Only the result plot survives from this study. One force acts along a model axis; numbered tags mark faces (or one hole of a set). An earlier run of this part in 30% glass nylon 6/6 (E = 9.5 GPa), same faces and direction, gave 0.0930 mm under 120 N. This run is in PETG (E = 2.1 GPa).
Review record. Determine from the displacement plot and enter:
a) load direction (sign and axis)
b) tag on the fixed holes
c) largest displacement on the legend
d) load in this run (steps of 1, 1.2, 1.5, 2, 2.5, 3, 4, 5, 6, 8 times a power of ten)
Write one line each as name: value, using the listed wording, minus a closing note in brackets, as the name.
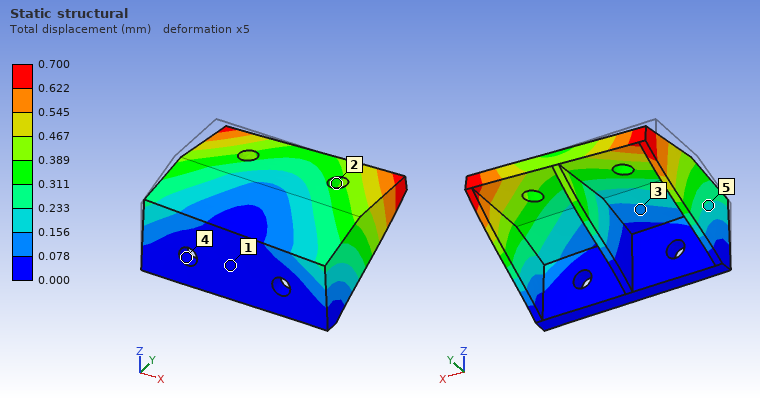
load direction: +X
tag on the fixed holes: 4
largest displacement on the legend: 0.700 mm
load in this run: 200 N
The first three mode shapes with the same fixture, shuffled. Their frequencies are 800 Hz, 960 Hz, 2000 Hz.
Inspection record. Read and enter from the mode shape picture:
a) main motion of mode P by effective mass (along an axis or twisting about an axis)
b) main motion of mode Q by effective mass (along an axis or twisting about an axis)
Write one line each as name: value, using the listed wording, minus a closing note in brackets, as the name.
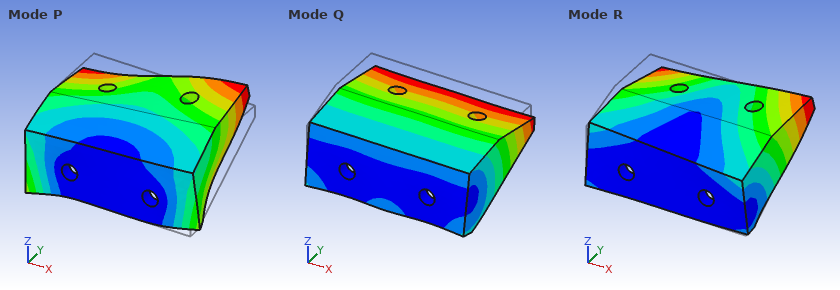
main motion of mode P by effective mass: along X
main motion of mode Q by effective mass: along Z
